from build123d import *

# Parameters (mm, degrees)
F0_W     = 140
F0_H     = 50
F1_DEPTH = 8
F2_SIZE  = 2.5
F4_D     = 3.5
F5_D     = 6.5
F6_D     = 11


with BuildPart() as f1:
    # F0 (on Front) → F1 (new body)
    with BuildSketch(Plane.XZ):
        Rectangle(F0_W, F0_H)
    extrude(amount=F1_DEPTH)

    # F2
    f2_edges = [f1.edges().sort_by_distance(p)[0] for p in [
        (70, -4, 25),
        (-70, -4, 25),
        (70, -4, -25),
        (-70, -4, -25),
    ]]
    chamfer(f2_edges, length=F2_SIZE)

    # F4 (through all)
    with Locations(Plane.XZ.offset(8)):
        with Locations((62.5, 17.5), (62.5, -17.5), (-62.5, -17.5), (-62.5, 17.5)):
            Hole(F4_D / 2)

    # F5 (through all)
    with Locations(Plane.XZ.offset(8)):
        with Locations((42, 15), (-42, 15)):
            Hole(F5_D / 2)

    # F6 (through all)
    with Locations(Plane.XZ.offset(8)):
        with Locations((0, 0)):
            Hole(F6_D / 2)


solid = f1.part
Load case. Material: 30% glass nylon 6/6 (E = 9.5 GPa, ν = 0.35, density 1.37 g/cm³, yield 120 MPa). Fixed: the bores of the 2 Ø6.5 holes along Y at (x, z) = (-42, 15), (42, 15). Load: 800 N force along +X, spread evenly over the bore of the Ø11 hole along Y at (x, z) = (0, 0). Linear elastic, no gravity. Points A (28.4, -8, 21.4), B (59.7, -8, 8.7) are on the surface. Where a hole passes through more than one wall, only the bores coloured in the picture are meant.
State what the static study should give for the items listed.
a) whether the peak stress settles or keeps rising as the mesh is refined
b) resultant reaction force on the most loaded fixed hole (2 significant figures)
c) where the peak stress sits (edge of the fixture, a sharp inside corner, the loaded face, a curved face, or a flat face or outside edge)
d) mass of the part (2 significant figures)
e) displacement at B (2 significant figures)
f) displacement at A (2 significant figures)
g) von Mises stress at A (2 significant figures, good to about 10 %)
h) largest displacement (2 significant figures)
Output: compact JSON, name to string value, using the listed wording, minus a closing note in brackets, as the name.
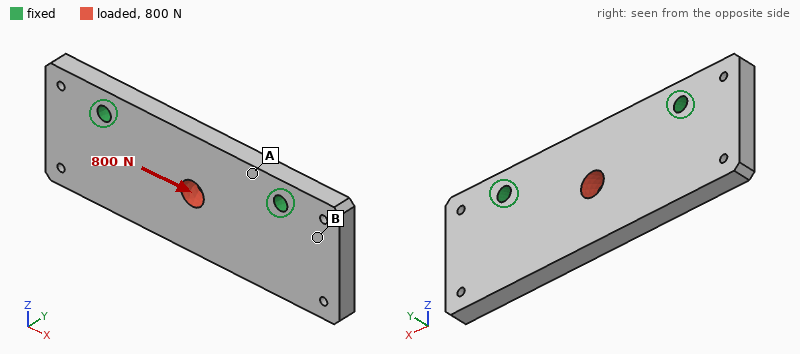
{"whether the peak stress settles or keeps rising as the mesh is refined": "keeps rising", "resultant reaction force on the most loaded fixed hole": "420 N", "where the peak stress sits": "edge of the fixture", "mass of the part": "74 g", "displacement at B": "4.6 µm", "displacement at A": "2.6 µm", "von Mises stress at A": "1.5 MPa", "largest displacement": "12 µm"}
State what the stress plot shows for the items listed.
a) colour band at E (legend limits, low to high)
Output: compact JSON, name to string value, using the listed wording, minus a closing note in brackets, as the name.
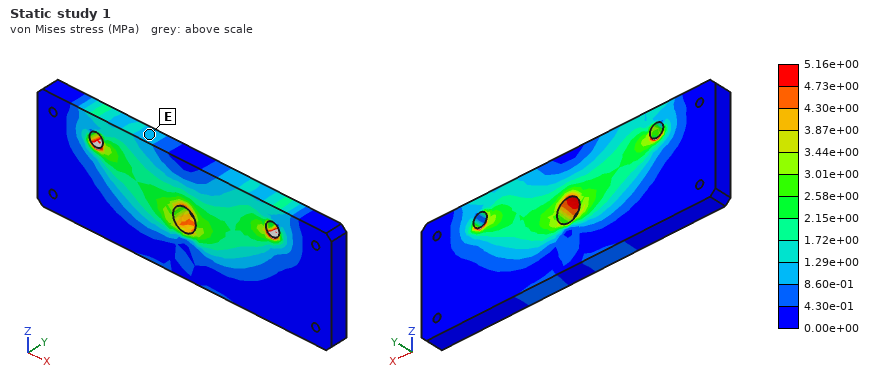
{"colour band at E": "8.60e-01 to 1.29e+00 MPa"}
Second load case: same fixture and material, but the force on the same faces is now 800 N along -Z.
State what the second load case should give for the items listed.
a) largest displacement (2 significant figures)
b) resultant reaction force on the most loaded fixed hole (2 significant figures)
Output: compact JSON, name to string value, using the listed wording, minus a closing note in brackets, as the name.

{"largest displacement": "24 µm", "resultant reaction force on the most loaded fixed hole": "470 N"}
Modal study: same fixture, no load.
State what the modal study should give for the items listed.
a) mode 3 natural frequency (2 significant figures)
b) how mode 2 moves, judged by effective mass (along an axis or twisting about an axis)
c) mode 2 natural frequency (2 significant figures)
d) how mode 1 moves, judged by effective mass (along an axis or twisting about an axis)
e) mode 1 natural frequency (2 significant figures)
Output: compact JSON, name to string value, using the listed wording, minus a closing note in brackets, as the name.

{"mode 3 natural frequency": "2200 Hz", "how mode 2 moves, judged by effective mass": "twisting about Z", "mode 2 natural frequency": "2000 Hz", "how mode 1 moves, judged by effective mass": "along Y", "mode 1 natural frequency": "1500 Hz"}
